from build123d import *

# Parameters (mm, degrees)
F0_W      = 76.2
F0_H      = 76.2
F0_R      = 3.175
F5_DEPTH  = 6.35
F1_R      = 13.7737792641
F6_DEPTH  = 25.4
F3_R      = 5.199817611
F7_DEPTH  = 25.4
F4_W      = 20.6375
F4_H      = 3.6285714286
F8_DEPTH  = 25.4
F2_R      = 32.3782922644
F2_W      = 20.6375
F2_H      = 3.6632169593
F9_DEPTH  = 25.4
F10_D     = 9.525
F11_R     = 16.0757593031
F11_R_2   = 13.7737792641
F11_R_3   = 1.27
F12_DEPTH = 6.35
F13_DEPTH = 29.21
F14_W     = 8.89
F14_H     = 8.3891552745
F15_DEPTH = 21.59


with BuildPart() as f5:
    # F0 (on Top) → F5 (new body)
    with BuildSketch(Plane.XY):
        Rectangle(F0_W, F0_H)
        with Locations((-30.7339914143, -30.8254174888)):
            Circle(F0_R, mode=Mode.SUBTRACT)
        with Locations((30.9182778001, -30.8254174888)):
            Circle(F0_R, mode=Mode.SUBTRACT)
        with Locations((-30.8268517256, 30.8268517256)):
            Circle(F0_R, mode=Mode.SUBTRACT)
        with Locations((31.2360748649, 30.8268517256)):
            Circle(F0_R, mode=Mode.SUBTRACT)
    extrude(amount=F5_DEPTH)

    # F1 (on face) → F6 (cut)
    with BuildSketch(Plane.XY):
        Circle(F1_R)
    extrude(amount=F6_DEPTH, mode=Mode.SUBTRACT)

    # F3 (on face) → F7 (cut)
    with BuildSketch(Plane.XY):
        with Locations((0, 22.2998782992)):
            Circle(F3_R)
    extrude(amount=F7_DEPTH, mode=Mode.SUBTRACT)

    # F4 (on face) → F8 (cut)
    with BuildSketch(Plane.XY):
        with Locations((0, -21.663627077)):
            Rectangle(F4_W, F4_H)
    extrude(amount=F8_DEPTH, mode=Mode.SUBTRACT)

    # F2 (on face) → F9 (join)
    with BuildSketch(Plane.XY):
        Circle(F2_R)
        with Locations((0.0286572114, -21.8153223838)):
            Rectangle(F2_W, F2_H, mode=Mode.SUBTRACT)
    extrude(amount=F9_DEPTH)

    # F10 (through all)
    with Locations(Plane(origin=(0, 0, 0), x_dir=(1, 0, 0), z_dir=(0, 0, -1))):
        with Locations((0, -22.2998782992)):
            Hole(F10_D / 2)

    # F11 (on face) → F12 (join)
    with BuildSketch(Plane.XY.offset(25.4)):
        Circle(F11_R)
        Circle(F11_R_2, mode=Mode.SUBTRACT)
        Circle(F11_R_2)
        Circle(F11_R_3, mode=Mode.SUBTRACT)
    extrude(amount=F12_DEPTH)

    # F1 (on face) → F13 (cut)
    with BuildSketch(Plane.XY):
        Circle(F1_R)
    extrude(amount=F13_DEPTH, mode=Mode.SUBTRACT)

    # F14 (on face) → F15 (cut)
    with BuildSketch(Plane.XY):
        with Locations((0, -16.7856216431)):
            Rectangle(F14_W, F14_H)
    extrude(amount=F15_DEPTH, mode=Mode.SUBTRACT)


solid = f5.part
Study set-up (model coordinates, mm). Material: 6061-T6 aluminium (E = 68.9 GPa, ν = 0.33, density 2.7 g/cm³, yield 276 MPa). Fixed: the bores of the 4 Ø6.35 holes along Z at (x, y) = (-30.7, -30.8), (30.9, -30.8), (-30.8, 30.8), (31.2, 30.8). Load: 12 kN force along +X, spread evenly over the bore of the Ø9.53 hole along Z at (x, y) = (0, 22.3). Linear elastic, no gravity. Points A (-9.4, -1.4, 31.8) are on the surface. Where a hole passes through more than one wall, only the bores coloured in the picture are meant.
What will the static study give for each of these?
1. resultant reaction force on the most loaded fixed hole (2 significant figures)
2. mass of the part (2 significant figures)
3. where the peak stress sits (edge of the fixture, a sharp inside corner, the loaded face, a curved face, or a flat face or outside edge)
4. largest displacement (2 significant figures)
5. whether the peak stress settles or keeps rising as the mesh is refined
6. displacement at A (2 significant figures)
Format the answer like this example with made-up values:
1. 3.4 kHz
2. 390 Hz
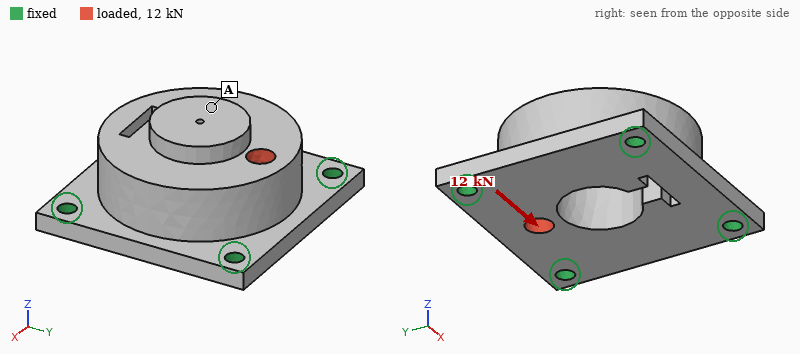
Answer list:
1. 5.1 kN
2. 220 g
3. edge of the fixture
4. 27 µm
5. keeps rising
6. 19 µm
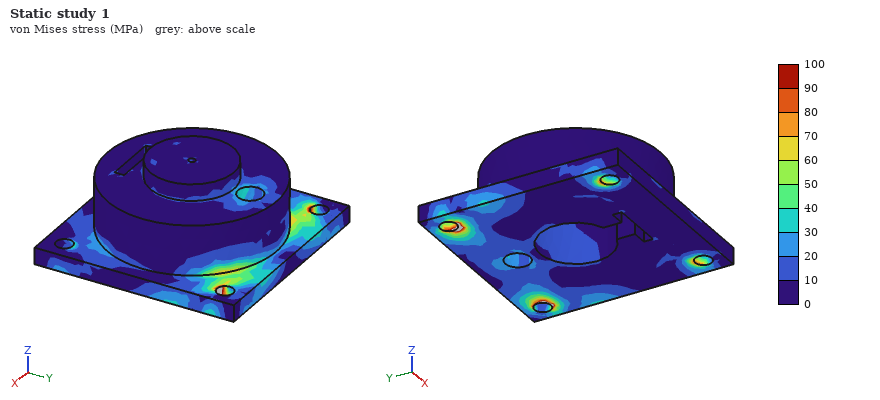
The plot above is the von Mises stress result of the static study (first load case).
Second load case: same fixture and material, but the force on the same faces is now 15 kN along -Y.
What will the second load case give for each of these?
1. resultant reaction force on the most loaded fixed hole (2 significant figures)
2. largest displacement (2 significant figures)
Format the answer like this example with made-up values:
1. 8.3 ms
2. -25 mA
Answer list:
1. 4.3 kN
2. 40 µm
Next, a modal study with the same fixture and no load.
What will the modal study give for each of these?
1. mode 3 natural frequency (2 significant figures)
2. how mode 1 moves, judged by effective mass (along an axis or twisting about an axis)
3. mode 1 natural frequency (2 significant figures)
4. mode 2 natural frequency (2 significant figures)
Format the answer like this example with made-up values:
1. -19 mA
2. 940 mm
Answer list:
1. 8200 Hz
2. along Z
3. 6700 Hz
4. 7900 Hz
